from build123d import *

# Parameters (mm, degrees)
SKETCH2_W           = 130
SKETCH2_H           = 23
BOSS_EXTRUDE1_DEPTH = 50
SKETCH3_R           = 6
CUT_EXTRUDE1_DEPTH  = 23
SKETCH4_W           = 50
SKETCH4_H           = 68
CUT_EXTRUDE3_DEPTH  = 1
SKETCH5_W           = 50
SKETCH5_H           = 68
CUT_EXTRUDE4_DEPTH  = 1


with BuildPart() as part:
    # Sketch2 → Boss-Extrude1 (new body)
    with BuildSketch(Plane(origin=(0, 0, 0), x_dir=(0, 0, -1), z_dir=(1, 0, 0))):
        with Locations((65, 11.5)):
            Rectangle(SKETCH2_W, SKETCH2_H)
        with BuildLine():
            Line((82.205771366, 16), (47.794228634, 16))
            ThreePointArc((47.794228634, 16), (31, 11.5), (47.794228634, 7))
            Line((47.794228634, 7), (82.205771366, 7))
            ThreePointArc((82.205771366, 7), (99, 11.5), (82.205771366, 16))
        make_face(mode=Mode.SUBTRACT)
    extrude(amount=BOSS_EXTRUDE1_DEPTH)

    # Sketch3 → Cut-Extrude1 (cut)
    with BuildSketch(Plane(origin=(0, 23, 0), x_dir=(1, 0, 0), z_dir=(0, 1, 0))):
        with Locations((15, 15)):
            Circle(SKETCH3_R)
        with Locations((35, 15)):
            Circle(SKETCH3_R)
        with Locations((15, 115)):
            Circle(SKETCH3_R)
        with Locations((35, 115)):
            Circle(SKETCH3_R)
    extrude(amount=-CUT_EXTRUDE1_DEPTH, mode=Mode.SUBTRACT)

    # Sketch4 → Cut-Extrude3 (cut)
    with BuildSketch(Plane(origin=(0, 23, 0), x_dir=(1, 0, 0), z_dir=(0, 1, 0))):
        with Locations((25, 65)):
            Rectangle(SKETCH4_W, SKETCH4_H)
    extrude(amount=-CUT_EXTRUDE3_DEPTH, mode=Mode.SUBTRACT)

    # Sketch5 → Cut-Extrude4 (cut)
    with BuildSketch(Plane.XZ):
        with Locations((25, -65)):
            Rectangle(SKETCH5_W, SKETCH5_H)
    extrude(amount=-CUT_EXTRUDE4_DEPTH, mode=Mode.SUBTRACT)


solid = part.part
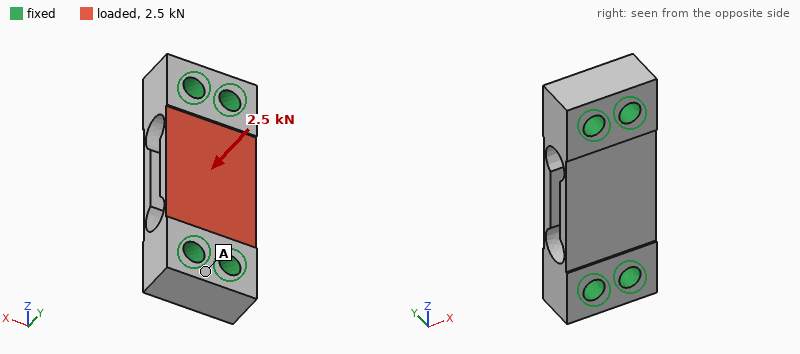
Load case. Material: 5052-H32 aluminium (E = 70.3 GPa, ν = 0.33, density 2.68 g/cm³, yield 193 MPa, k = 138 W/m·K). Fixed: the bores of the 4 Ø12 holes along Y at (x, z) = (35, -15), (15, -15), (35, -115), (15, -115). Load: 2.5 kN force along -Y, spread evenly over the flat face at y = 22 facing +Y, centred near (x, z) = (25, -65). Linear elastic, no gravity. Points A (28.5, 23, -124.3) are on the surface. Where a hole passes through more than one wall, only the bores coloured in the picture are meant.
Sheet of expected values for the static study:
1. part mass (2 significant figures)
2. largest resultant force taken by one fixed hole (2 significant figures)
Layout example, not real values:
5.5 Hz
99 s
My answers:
250 g
720 N
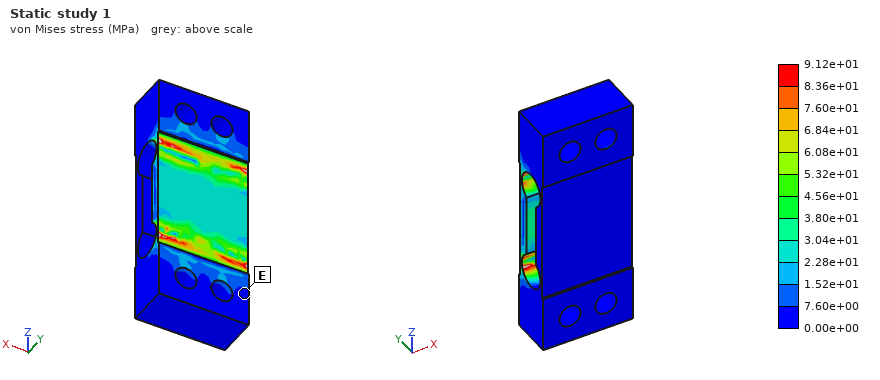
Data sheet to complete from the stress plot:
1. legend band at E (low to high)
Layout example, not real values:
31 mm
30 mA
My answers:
0.00e+00 to 7.60e+00 MPa
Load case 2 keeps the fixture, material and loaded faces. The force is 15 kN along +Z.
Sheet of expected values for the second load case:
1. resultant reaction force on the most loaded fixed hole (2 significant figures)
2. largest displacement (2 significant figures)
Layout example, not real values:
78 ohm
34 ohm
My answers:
3.8 kN
25 µm
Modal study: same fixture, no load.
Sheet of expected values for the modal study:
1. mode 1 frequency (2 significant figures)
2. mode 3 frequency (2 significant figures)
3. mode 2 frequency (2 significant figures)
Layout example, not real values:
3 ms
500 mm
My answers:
4200 Hz
4600 Hz
4300 Hz
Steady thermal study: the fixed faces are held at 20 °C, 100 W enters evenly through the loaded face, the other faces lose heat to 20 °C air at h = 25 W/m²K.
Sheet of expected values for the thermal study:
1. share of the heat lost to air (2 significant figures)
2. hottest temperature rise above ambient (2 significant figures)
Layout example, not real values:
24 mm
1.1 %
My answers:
4.6 %
50 K
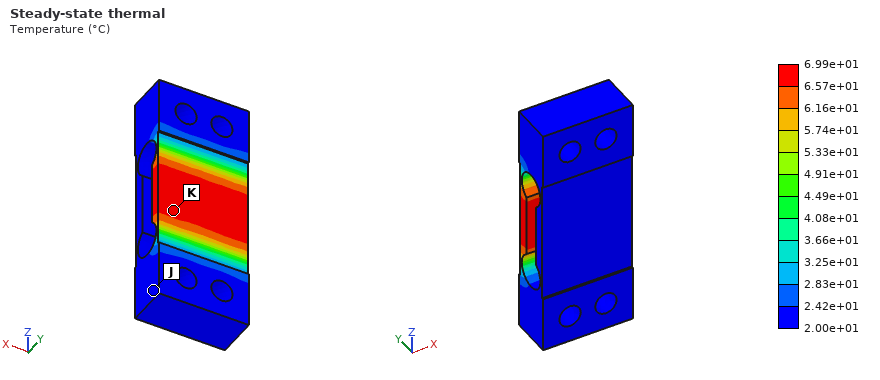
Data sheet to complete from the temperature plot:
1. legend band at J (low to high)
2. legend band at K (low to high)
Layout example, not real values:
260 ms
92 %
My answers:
2.00e+01 to 2.42e+01 °C
6.57e+01 to 6.99e+01 °C
